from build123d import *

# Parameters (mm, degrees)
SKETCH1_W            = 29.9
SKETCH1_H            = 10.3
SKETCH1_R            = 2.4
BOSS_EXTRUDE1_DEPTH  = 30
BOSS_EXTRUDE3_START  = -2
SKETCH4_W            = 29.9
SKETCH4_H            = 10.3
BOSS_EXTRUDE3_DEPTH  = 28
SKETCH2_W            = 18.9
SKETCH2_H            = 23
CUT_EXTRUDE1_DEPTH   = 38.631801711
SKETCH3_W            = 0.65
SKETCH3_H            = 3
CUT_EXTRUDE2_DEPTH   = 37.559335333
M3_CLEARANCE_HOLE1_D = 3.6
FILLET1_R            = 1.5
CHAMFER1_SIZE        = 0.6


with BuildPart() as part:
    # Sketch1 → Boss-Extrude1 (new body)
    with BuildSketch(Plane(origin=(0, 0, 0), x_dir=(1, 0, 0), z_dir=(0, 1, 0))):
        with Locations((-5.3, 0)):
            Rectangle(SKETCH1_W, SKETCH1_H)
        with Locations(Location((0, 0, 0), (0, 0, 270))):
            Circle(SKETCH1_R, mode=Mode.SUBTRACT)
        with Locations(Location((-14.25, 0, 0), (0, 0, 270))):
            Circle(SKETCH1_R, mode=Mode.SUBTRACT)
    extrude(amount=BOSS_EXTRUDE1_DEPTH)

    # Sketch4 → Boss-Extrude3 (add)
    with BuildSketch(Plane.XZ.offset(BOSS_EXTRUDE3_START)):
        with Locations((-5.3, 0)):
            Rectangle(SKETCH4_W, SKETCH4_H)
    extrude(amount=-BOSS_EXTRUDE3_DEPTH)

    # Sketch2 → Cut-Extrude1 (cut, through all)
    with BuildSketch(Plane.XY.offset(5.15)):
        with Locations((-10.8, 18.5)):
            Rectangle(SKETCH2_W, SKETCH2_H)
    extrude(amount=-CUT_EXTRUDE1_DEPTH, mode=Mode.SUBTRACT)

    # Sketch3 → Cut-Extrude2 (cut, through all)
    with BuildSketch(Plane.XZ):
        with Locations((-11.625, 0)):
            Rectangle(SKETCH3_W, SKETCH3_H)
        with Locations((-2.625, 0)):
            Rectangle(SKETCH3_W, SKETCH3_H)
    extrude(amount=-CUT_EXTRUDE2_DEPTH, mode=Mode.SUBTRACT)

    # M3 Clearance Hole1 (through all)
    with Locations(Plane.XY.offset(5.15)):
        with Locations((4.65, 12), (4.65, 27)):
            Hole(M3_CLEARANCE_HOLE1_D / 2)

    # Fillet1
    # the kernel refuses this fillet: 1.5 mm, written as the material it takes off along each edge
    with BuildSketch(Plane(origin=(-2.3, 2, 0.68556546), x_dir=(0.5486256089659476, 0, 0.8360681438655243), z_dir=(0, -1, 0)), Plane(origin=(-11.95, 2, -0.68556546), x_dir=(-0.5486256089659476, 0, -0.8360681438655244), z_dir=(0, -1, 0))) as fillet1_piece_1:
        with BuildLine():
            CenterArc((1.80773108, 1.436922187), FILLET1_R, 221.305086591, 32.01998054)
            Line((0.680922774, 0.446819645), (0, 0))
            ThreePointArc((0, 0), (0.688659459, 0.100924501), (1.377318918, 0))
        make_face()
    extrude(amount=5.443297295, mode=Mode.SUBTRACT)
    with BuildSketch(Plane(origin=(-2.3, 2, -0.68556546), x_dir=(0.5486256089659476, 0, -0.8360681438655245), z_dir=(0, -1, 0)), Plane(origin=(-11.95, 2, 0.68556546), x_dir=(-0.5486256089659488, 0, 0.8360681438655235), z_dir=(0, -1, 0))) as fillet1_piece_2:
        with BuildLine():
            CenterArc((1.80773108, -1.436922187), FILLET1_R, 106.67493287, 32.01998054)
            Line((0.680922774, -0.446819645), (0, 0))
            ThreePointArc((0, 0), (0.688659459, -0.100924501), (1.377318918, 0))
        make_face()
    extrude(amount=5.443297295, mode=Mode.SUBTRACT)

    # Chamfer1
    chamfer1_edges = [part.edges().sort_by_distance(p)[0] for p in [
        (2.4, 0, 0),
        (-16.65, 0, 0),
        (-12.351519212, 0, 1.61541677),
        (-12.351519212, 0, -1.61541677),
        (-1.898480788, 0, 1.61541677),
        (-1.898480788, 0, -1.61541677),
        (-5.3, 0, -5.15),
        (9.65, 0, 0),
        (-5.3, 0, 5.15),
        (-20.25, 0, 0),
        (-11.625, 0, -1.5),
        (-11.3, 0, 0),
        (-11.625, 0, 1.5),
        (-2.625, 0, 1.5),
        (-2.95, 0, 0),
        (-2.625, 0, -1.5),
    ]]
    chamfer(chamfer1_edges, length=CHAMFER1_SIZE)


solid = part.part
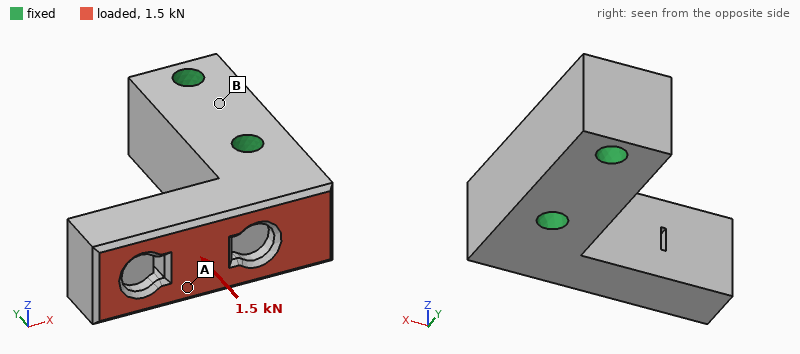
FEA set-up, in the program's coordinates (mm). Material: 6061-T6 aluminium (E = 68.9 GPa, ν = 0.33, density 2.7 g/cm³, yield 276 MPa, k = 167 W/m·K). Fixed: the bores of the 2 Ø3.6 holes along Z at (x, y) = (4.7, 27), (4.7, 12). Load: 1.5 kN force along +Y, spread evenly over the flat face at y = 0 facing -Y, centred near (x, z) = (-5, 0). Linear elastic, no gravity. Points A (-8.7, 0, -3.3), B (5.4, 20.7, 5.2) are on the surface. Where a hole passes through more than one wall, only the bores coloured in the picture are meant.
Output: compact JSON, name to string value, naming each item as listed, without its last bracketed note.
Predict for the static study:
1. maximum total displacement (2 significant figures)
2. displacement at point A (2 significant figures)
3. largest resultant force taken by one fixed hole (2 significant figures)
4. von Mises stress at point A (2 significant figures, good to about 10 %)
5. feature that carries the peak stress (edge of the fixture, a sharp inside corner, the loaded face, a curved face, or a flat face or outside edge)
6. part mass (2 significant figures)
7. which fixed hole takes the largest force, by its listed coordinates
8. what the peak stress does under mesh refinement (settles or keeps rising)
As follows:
{"maximum total displacement": "0.14 mm", "displacement at point A": "0.067 mm", "largest resultant force taken by one fixed hole": "1.3 kN", "von Mises stress at point A": "43 MPa", "feature that carries the peak stress": "a sharp inside corner", "part mass": "12 g", "which fixed hole takes the largest force, by its listed coordinates": "(4.7, 12)", "what the peak stress does under mesh refinement": "keeps rising"}
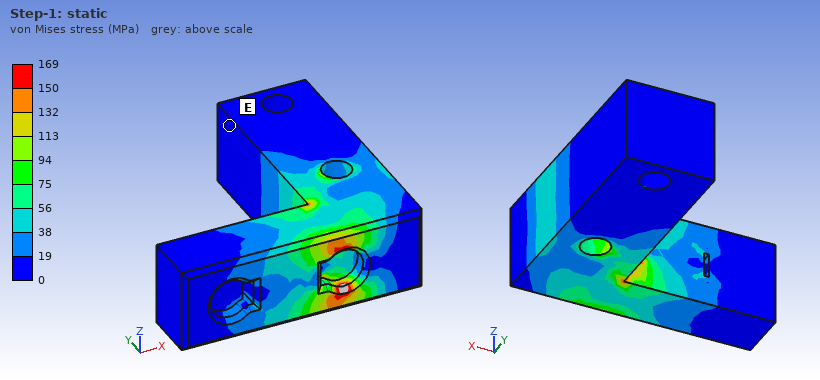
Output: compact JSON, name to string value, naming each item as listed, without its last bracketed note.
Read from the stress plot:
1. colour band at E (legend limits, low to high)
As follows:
{"colour band at E": "0 to 19 MPa"}
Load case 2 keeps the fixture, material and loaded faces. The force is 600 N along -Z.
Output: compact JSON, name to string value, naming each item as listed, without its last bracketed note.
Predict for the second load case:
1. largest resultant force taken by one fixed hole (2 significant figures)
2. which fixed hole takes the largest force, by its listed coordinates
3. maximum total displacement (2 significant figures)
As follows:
{"largest resultant force taken by one fixed hole": "650 N", "which fixed hole takes the largest force, by its listed coordinates": "(4.7, 12)", "maximum total displacement": "43 µm"}
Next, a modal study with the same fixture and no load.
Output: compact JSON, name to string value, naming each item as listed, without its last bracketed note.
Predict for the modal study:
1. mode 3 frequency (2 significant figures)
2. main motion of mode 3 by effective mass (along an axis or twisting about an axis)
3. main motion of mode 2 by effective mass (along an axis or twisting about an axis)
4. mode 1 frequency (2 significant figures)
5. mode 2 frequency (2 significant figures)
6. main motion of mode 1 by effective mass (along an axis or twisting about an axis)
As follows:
{"mode 3 frequency": "26 kHz", "main motion of mode 3 by effective mass": "along X", "main motion of mode 2 by effective mass": "along Z", "mode 1 frequency": "8200 Hz", "mode 2 frequency": "10 kHz", "main motion of mode 1 by effective mass": "along Y"}
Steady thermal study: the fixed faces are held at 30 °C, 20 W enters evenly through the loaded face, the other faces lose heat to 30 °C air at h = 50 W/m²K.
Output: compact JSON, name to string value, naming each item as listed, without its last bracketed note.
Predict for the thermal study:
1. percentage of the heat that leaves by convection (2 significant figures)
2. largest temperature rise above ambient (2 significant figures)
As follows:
{"percentage of the heat that leaves by convection": "3.7 %", "largest temperature rise above ambient": "22 K"}
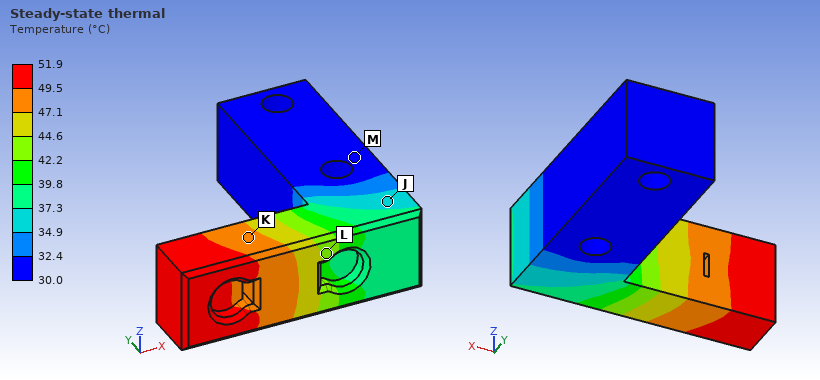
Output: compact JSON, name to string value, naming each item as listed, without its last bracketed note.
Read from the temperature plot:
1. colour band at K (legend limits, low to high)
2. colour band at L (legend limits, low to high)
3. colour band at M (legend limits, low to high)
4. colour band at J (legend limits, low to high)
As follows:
{"colour band at K": "47.1 to 49.5 °C", "colour band at L": "42.2 to 44.6 °C", "colour band at M": "30.0 to 32.4 °C", "colour band at J": "34.9 to 37.3 °C"}
